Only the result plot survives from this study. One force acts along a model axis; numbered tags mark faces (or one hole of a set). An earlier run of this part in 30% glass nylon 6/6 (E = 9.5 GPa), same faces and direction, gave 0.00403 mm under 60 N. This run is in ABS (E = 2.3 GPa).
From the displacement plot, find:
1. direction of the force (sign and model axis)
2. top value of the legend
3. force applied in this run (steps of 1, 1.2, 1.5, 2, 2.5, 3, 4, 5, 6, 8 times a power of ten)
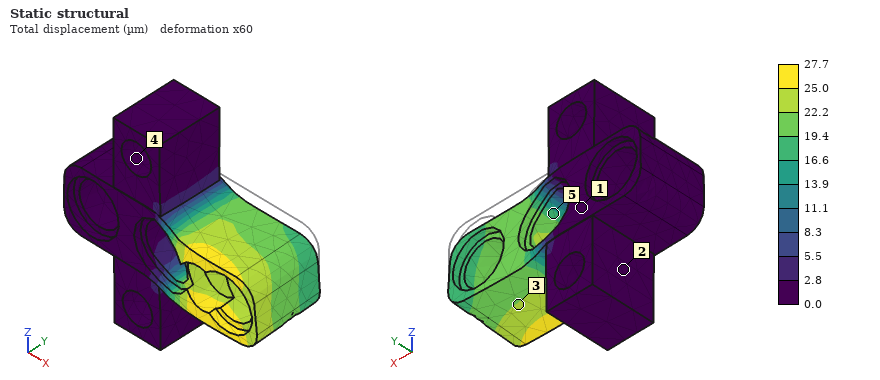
-Z
27.7 µm
100 N
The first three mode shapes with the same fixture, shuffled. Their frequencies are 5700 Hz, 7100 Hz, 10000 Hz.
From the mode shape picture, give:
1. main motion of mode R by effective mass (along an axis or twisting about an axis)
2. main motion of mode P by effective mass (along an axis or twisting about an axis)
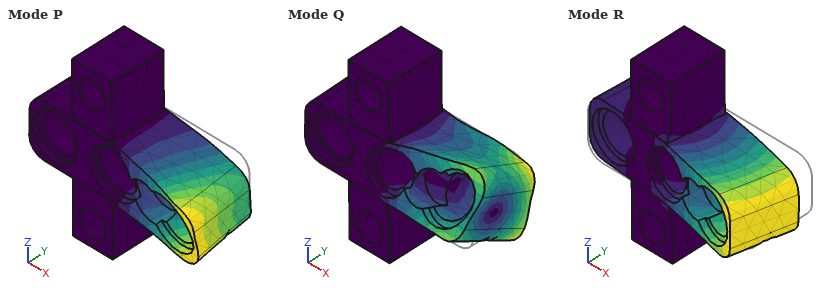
along Y
along Z
